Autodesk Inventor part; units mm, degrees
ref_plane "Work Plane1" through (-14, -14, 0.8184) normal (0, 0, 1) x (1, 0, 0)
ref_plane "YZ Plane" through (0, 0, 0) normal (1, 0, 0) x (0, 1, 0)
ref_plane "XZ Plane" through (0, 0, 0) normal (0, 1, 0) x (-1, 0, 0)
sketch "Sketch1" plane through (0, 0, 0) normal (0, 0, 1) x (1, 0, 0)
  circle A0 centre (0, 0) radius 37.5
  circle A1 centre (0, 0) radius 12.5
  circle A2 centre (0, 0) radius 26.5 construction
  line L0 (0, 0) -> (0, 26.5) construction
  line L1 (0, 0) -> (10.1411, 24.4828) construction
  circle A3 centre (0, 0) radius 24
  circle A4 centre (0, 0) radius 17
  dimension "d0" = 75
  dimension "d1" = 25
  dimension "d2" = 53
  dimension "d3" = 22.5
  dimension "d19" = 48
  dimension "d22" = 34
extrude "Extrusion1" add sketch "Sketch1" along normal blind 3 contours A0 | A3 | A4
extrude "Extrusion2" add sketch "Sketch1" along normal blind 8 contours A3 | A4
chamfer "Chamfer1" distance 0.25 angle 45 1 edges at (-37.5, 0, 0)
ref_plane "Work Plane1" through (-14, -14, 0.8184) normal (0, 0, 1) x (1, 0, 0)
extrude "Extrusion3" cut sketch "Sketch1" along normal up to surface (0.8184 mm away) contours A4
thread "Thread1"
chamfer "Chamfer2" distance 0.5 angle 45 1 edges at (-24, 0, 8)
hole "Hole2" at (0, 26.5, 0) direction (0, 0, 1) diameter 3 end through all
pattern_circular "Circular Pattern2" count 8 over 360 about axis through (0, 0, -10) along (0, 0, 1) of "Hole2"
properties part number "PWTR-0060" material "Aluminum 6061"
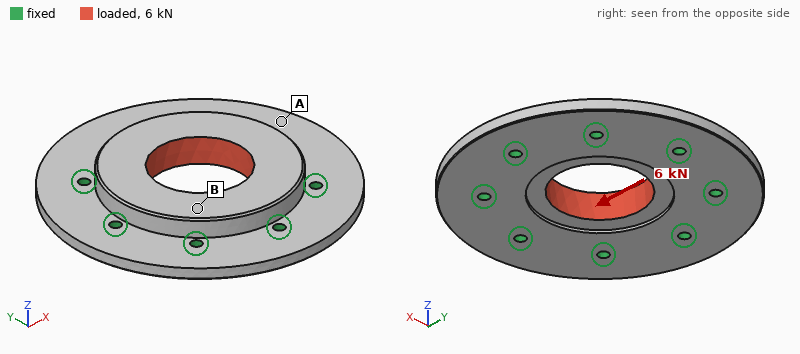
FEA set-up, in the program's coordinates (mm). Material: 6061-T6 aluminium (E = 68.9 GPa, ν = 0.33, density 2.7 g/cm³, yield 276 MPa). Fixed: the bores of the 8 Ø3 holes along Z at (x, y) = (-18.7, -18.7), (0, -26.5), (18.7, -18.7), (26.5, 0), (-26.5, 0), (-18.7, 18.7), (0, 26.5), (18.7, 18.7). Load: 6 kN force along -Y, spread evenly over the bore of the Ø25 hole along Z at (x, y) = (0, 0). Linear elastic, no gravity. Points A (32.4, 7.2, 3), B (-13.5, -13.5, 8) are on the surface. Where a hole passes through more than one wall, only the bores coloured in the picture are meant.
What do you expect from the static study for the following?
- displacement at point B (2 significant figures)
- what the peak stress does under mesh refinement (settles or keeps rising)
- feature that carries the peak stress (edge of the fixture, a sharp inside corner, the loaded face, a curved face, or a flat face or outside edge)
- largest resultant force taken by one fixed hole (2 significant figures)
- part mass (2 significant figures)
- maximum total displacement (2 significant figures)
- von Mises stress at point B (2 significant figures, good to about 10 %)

4.6 µm
keeps rising
edge of the fixture
1.0 kN
48 g
8.4 µm
10 MPa
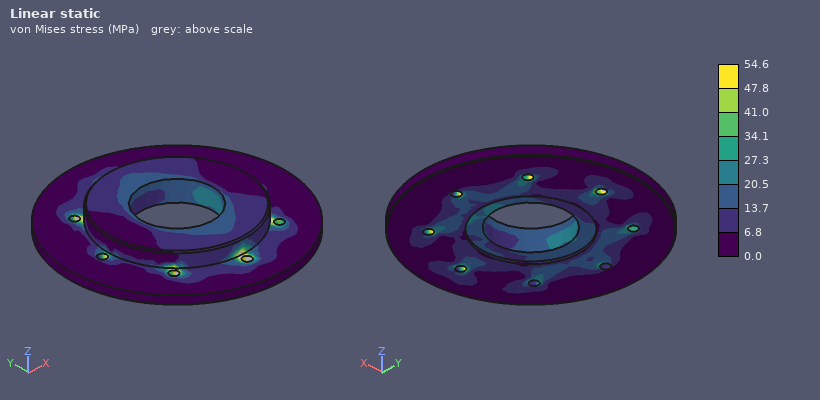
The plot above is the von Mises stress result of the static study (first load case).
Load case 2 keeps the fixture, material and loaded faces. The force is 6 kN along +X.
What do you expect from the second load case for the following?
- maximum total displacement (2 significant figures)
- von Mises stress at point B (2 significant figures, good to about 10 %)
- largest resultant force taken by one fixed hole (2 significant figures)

8.4 µm
10.0 MPa
1.0 kN
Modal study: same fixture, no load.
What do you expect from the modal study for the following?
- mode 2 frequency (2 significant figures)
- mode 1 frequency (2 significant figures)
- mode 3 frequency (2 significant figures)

16 kHz
16 kHz
16 kHz
